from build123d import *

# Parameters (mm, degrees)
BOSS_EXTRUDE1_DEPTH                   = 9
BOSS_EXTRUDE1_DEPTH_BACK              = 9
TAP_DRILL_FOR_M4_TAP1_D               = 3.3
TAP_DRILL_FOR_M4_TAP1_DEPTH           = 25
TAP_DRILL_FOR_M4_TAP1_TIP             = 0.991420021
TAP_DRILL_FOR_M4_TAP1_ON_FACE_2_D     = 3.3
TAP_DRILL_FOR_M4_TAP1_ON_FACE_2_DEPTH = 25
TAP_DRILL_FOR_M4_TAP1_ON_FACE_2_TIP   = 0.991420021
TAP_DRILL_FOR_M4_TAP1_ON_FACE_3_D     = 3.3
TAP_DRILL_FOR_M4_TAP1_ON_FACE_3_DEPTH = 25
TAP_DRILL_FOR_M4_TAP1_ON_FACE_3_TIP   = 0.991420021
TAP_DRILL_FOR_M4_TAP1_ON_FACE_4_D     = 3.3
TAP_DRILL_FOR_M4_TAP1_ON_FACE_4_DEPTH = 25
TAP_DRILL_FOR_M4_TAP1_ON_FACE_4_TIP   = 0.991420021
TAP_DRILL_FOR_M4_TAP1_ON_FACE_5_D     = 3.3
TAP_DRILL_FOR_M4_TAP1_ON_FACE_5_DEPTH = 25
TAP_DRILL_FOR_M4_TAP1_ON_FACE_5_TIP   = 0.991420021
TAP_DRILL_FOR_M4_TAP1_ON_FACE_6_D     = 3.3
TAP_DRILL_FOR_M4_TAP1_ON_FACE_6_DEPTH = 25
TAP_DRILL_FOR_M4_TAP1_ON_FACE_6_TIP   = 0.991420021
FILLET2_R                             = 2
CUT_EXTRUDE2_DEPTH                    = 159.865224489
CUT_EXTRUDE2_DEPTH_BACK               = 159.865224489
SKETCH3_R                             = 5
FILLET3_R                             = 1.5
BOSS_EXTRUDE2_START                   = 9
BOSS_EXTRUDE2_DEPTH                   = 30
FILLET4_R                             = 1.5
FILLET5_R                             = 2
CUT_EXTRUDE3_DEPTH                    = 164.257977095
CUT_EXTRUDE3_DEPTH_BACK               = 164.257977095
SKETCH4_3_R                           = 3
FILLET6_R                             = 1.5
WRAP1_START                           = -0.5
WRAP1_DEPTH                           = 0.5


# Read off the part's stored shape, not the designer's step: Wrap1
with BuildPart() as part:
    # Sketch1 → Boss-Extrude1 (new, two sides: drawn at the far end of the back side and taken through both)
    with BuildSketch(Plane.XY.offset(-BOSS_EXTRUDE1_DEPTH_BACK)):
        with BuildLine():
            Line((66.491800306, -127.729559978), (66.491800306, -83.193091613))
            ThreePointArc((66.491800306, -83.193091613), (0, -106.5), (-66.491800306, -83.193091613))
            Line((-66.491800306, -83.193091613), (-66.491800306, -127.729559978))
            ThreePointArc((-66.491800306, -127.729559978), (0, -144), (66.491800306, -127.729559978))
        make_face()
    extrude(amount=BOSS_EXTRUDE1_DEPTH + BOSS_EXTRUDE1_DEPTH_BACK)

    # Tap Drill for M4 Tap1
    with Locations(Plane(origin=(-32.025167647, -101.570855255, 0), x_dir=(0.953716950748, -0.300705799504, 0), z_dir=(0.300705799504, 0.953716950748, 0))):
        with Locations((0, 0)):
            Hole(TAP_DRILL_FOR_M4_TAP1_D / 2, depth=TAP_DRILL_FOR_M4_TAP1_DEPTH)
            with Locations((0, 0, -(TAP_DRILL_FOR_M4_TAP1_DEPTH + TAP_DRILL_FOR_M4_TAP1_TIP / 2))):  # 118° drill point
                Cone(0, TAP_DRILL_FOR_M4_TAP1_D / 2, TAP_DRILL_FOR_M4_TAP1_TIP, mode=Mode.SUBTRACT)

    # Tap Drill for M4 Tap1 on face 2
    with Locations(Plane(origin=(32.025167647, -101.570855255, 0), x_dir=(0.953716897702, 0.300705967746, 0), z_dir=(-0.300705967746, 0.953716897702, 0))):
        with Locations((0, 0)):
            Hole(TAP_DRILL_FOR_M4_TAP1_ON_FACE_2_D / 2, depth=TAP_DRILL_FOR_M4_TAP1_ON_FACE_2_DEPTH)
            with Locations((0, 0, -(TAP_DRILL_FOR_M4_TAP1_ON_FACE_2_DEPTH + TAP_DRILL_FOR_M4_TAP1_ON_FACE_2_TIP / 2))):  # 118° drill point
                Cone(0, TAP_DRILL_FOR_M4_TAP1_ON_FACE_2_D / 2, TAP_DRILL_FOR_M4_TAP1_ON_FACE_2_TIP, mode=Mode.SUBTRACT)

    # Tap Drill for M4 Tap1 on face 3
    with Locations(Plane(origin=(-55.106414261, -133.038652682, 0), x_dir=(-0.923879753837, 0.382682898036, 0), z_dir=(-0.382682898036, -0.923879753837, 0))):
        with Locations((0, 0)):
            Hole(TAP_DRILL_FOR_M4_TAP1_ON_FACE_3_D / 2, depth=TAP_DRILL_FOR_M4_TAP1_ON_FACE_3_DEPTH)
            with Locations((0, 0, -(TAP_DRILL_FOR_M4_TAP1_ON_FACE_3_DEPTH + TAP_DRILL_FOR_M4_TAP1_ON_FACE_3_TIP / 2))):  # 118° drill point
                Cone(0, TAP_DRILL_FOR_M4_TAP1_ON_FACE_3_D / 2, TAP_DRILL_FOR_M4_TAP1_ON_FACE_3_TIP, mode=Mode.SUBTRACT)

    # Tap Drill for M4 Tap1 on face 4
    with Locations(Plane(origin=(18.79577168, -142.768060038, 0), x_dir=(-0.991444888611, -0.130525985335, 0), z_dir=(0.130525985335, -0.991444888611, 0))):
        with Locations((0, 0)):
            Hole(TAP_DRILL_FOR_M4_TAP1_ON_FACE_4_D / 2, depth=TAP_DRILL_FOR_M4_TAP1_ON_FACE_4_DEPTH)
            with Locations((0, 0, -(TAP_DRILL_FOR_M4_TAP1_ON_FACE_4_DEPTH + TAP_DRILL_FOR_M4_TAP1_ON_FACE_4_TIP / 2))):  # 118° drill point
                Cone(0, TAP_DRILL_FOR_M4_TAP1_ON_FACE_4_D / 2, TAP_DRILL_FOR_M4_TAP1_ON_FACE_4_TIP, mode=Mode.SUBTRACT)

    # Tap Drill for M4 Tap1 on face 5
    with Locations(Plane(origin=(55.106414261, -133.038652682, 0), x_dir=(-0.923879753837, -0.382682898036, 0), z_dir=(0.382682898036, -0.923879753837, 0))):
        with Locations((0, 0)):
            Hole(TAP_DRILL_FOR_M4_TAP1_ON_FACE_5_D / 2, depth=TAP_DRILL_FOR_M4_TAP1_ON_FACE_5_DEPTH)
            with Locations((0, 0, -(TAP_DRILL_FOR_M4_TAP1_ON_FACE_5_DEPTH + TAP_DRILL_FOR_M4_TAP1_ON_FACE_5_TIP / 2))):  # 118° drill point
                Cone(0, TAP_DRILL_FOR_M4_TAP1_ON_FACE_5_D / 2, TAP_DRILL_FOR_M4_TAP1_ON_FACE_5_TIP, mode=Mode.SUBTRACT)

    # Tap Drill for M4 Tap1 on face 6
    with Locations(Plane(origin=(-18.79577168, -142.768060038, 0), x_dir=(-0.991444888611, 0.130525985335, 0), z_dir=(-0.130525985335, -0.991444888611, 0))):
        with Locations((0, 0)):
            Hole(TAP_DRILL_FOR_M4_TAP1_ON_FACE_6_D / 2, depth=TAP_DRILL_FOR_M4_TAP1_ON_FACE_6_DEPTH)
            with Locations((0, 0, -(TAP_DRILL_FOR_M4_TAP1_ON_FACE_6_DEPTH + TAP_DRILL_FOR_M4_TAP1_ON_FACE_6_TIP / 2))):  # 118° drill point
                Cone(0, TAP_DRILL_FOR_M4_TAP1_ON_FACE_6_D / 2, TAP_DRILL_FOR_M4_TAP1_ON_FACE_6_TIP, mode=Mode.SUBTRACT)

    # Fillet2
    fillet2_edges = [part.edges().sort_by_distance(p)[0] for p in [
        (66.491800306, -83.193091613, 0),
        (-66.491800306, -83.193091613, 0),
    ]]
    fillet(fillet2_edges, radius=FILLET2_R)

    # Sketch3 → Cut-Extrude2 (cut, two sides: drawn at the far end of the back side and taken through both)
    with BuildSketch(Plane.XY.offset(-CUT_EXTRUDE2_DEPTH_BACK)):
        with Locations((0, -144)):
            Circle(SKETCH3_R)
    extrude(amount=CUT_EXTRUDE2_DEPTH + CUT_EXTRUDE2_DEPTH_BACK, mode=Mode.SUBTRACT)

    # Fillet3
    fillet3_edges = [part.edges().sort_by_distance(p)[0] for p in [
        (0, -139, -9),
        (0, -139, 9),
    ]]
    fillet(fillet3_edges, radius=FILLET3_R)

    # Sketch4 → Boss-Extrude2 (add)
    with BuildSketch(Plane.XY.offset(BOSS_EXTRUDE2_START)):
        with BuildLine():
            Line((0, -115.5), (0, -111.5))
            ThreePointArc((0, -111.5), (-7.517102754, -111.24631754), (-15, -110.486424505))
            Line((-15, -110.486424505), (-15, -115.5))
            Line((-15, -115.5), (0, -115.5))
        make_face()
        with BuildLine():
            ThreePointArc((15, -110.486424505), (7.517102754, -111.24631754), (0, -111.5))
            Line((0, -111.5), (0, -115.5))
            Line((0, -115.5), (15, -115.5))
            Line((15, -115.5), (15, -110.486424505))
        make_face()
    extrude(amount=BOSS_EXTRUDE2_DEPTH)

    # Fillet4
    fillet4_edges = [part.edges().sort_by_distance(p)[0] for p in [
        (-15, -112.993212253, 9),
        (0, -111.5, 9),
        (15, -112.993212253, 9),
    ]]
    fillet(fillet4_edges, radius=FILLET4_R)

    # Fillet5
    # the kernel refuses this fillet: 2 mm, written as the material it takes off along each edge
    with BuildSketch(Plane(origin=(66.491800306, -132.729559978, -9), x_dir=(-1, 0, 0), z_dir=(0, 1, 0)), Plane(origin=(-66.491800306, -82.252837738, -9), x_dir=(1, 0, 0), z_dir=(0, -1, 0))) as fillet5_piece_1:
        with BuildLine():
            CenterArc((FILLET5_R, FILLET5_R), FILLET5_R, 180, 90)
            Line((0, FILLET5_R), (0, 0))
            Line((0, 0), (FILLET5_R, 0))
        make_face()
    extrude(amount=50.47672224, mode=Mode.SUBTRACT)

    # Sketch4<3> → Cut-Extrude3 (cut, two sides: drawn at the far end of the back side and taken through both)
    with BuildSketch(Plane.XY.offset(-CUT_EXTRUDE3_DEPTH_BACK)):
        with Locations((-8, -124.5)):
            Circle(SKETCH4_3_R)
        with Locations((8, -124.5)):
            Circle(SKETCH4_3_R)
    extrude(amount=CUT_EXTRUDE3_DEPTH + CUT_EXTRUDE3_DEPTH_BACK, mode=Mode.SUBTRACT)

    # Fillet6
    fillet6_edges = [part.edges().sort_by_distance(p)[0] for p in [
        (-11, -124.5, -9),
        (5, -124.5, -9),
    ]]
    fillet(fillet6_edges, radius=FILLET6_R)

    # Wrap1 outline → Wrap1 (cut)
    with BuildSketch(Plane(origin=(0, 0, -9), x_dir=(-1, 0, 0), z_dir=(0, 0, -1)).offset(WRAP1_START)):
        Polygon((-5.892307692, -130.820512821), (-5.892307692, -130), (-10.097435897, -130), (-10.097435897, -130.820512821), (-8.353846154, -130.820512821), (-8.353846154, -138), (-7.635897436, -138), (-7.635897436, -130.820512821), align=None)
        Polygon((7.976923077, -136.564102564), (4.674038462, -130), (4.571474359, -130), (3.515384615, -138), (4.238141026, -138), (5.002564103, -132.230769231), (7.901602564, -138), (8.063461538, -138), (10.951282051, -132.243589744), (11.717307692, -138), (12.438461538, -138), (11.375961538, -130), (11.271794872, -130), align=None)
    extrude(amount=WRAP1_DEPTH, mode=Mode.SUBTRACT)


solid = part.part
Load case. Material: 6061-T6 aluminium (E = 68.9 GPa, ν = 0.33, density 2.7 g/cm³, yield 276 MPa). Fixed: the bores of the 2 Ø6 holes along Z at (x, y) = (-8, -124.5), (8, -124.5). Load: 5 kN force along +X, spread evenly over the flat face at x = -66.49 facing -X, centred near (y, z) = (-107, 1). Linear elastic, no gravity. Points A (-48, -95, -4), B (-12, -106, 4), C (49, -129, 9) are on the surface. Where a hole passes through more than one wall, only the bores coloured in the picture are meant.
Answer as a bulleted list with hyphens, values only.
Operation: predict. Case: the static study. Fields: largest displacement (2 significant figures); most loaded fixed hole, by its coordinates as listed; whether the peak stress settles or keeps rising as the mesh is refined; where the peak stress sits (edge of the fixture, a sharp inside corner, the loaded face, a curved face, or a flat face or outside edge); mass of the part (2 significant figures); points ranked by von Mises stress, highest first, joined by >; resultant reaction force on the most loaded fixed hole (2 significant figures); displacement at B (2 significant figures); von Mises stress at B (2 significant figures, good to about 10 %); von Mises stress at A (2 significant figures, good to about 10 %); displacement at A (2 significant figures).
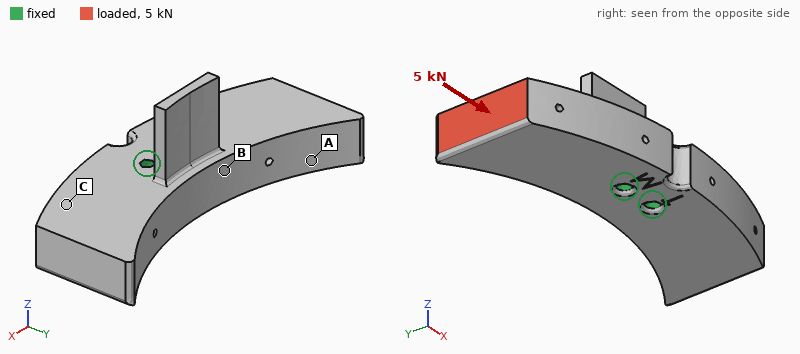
- 68 µm
- (-8, -124.5)
- keeps rising
- edge of the fixture
- 260 g
- B > A > C
- 5.0 kN
- 11 µm
- 29 MPa
- 14 MPa
- 43 µm
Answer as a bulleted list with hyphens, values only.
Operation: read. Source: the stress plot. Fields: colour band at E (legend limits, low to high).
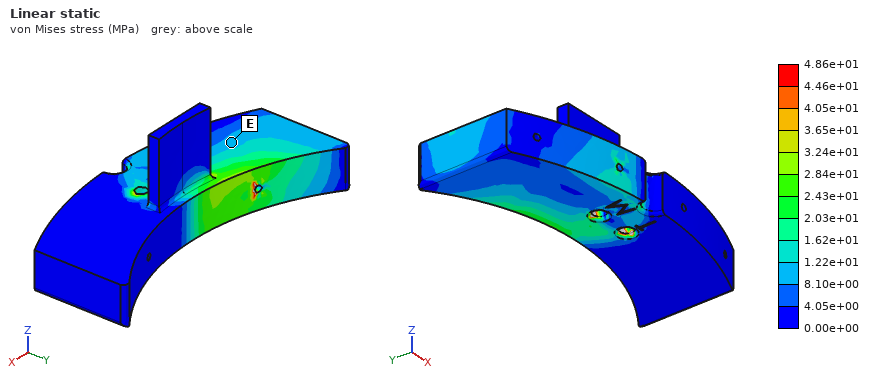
- 8.10e+00 to 1.22e+01 MPa
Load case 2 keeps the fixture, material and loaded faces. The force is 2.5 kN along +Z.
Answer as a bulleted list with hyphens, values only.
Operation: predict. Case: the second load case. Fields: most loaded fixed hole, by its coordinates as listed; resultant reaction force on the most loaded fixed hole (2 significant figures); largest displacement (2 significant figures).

- (-8, -124.5)
- 4.9 kN
- 0.22 mm
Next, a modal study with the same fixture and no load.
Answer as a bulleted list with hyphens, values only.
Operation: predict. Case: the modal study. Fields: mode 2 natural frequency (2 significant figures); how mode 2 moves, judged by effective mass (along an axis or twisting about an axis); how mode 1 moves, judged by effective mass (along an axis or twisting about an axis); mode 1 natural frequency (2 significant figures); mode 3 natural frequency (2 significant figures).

- 3400 Hz
- along Z
- twisting about Y
- 3200 Hz
- 3800 Hz
